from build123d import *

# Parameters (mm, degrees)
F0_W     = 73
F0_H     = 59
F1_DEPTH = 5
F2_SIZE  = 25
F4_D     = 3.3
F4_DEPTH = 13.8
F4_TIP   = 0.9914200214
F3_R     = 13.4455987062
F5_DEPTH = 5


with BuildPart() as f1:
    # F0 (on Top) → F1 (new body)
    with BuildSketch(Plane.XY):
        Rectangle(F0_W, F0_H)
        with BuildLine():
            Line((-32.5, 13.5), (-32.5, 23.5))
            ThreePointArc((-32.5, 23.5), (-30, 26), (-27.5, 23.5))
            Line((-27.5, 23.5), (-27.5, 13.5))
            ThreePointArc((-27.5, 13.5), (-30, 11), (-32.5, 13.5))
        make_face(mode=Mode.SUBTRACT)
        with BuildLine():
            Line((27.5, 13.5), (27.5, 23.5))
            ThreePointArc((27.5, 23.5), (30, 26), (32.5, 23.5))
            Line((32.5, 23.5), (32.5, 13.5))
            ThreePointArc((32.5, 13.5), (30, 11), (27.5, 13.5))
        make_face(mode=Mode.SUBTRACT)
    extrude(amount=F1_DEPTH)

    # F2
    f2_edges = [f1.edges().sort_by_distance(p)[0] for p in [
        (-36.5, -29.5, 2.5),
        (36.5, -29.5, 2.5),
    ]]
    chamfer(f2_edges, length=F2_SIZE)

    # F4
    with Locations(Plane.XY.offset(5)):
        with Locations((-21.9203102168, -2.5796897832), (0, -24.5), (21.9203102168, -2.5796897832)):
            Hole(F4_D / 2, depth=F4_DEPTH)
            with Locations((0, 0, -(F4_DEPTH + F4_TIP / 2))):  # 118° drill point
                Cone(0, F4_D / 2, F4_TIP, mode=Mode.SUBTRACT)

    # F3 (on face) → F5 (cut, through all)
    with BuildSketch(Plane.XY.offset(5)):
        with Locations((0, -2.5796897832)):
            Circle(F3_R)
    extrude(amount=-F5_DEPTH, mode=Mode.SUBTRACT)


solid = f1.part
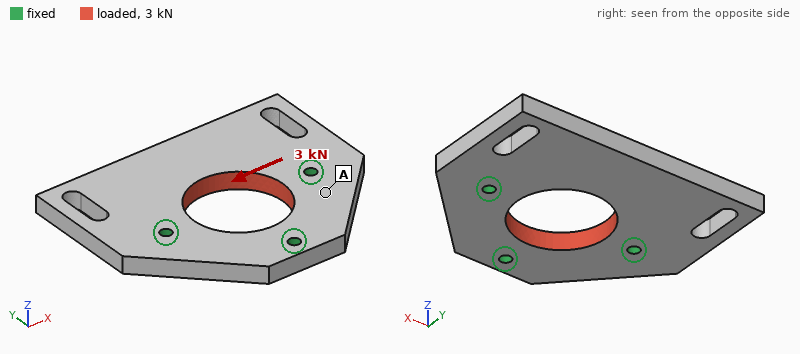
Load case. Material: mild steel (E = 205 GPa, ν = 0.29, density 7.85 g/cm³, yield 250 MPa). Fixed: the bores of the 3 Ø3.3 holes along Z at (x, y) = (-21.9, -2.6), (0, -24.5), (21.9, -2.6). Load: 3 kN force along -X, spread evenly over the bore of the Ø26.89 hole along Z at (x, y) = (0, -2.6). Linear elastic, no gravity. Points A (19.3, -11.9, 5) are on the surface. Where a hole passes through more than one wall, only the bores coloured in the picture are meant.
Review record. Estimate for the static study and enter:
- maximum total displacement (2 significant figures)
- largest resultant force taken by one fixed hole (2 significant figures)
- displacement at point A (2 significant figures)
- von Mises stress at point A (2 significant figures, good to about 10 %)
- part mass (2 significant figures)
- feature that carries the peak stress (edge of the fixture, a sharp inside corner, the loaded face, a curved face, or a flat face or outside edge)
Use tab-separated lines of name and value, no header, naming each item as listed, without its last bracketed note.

maximum total displacement	2.4 µm
largest resultant force taken by one fixed hole	1.2 kN
displacement at point A	0.49 µm
von Mises stress at point A	7.5 MPa
part mass	120 g
feature that carries the peak stress	edge of the fixture
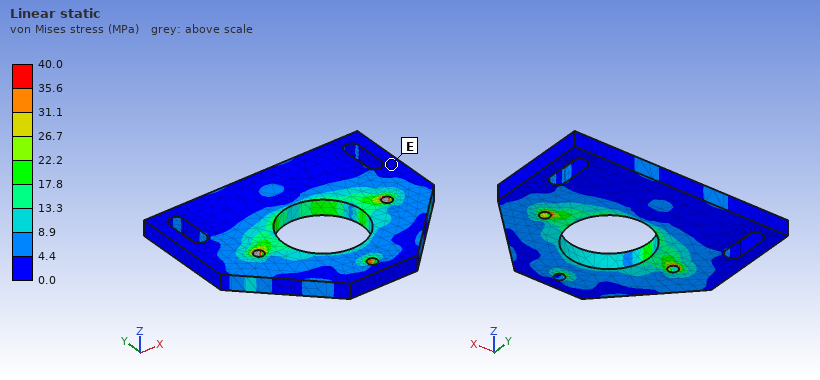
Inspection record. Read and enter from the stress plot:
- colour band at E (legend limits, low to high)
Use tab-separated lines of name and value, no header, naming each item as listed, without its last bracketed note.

colour band at E	0.0 to 4.4 MPa
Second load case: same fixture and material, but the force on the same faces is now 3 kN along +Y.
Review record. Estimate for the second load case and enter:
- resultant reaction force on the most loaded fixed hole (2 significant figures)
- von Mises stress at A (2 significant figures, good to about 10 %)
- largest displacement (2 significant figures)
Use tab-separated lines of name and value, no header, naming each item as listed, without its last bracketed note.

resultant reaction force on the most loaded fixed hole	1.1 kN
von Mises stress at A	7.4 MPa
largest displacement	1.9 µm
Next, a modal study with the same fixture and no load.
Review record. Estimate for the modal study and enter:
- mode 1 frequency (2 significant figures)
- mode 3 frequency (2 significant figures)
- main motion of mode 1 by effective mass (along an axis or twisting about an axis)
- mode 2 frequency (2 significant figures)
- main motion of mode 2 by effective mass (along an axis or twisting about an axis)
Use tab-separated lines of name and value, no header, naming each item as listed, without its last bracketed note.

mode 1 frequency	3000 Hz
mode 3 frequency	7900 Hz
main motion of mode 1 by effective mass	along Z
mode 2 frequency	5000 Hz
main motion of mode 2 by effective mass	twisting about Y
